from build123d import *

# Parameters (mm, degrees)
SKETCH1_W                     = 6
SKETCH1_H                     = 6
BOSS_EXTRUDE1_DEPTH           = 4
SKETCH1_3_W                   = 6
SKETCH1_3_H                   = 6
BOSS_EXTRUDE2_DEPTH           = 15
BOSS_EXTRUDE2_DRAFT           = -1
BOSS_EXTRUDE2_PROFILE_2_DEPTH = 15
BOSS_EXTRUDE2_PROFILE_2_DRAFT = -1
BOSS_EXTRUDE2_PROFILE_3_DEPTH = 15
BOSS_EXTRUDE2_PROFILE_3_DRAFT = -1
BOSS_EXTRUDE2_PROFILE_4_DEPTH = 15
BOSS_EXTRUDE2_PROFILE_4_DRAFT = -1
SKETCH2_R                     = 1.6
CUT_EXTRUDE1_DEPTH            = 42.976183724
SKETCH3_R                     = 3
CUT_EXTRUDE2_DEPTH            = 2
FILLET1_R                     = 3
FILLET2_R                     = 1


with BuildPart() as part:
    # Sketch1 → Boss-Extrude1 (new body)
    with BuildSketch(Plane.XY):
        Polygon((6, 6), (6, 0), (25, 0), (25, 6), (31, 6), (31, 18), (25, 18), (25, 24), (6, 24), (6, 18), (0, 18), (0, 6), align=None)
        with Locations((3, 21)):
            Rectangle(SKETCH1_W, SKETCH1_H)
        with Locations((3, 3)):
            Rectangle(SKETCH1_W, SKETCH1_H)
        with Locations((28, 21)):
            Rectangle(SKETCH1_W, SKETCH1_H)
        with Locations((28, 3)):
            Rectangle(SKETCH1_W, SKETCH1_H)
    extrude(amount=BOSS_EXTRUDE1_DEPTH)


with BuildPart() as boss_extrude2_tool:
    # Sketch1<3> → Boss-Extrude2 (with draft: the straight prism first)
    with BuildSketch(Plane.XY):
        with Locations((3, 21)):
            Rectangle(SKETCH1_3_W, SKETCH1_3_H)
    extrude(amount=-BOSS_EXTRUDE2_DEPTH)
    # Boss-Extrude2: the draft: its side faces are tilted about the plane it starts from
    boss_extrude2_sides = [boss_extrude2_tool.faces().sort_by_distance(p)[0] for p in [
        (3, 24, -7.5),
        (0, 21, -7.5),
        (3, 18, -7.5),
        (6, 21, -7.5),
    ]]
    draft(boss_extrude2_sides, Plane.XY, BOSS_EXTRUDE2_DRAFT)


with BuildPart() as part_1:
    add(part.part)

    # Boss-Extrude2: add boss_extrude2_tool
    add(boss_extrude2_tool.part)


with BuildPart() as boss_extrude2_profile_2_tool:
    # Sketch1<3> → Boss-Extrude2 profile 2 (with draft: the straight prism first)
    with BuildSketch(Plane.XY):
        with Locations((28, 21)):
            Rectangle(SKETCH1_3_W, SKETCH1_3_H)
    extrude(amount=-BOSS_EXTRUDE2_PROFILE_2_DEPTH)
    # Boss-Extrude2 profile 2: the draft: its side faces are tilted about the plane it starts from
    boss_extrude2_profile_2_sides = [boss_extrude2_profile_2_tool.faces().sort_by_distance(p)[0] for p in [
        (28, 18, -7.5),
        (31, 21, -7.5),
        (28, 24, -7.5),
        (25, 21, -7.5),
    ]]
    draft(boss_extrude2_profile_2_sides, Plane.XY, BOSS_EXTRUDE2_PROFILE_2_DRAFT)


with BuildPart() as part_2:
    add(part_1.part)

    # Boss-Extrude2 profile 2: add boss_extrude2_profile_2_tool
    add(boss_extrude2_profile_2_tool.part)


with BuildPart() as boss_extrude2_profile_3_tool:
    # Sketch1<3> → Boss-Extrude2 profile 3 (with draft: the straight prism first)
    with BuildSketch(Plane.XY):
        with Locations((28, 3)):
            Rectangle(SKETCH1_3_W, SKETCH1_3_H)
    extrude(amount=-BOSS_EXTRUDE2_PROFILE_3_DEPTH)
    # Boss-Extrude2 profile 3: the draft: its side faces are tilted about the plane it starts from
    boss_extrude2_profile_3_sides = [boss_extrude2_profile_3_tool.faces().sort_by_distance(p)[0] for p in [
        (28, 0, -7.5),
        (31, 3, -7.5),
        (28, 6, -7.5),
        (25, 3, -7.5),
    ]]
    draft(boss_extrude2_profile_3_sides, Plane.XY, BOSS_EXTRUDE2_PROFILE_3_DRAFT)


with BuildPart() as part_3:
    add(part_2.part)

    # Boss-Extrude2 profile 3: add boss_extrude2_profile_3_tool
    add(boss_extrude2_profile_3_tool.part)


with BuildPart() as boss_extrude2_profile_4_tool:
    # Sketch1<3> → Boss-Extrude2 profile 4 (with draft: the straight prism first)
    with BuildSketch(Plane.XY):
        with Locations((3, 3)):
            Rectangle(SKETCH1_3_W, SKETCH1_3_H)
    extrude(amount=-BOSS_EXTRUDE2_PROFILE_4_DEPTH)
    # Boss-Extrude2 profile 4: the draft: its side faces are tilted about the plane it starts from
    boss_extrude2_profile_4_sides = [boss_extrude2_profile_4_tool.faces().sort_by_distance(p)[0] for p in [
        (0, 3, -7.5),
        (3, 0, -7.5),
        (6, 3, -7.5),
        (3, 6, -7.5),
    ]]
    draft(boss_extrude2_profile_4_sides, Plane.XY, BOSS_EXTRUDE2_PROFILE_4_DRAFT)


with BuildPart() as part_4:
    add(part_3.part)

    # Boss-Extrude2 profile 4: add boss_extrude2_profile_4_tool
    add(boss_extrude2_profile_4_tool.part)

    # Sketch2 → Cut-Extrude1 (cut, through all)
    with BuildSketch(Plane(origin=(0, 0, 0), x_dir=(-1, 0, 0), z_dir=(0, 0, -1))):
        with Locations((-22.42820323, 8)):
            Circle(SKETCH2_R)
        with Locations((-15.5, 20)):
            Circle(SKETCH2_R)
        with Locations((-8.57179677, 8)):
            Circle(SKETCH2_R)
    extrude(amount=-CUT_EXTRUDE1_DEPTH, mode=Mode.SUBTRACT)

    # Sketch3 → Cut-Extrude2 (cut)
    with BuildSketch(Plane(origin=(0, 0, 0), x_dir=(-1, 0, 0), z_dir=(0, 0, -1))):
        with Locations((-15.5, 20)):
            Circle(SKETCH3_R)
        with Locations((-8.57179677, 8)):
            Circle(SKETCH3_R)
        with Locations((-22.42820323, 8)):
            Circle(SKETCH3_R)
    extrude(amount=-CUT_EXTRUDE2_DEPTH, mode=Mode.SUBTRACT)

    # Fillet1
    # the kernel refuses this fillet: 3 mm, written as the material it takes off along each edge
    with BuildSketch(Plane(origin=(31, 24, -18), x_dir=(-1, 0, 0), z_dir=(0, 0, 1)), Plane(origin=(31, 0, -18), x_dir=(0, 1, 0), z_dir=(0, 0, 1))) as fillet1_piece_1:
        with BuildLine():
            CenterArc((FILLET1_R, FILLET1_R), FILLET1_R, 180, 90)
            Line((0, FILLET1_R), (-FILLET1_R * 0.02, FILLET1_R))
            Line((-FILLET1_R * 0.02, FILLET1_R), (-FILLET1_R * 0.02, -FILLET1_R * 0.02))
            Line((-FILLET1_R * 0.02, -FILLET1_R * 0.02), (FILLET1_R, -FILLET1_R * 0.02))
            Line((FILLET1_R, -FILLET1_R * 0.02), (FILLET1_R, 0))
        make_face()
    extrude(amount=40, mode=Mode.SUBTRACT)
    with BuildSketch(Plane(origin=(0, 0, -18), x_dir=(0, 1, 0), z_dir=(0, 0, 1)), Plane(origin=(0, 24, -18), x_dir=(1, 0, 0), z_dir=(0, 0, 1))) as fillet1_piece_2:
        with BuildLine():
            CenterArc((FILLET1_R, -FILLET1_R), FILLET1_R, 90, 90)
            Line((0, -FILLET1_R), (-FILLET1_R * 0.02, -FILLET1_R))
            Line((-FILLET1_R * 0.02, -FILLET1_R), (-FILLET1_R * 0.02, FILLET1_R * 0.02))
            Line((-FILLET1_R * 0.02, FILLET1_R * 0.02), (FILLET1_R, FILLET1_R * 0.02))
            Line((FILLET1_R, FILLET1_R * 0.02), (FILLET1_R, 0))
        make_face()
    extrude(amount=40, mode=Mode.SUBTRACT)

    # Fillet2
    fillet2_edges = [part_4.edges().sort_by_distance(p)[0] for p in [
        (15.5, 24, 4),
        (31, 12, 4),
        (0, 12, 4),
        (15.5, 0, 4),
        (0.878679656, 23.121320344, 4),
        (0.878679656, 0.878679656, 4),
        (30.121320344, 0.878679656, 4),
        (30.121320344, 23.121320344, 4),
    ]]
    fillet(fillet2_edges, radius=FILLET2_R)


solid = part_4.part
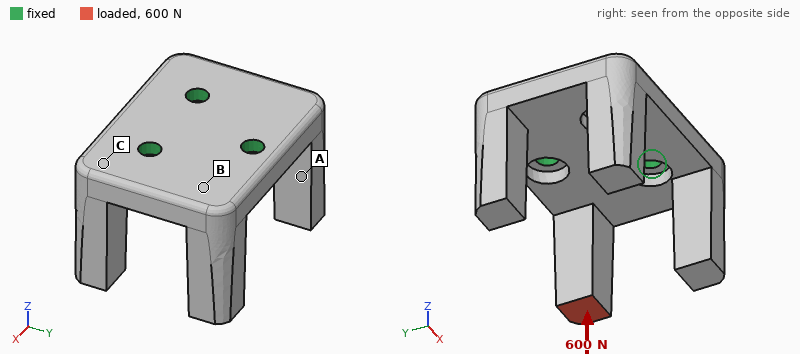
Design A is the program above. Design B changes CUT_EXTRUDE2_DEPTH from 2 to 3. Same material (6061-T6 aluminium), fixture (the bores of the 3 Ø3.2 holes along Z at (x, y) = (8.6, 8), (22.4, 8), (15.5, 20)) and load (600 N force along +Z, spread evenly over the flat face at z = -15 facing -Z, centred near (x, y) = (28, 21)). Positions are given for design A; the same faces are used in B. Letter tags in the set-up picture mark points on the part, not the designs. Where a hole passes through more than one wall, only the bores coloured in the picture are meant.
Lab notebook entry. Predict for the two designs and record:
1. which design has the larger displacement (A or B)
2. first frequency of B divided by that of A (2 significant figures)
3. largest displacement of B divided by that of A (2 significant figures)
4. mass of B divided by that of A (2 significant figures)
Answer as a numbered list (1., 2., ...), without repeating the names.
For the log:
1. B
2. 0.89
3. 1.2
4. 0.99
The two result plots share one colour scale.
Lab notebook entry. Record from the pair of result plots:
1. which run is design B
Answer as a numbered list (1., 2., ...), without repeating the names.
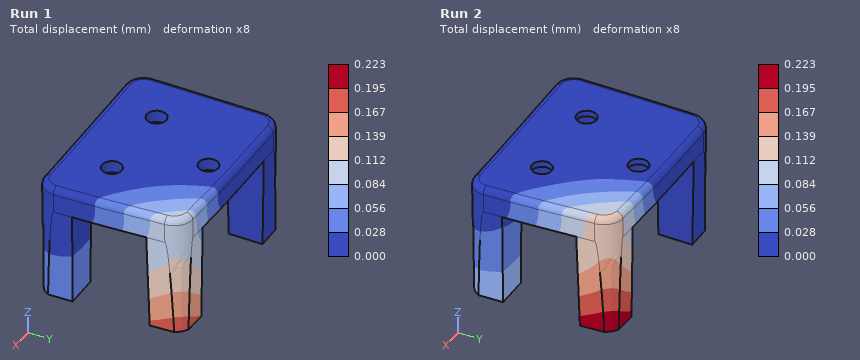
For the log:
1. Run 2
